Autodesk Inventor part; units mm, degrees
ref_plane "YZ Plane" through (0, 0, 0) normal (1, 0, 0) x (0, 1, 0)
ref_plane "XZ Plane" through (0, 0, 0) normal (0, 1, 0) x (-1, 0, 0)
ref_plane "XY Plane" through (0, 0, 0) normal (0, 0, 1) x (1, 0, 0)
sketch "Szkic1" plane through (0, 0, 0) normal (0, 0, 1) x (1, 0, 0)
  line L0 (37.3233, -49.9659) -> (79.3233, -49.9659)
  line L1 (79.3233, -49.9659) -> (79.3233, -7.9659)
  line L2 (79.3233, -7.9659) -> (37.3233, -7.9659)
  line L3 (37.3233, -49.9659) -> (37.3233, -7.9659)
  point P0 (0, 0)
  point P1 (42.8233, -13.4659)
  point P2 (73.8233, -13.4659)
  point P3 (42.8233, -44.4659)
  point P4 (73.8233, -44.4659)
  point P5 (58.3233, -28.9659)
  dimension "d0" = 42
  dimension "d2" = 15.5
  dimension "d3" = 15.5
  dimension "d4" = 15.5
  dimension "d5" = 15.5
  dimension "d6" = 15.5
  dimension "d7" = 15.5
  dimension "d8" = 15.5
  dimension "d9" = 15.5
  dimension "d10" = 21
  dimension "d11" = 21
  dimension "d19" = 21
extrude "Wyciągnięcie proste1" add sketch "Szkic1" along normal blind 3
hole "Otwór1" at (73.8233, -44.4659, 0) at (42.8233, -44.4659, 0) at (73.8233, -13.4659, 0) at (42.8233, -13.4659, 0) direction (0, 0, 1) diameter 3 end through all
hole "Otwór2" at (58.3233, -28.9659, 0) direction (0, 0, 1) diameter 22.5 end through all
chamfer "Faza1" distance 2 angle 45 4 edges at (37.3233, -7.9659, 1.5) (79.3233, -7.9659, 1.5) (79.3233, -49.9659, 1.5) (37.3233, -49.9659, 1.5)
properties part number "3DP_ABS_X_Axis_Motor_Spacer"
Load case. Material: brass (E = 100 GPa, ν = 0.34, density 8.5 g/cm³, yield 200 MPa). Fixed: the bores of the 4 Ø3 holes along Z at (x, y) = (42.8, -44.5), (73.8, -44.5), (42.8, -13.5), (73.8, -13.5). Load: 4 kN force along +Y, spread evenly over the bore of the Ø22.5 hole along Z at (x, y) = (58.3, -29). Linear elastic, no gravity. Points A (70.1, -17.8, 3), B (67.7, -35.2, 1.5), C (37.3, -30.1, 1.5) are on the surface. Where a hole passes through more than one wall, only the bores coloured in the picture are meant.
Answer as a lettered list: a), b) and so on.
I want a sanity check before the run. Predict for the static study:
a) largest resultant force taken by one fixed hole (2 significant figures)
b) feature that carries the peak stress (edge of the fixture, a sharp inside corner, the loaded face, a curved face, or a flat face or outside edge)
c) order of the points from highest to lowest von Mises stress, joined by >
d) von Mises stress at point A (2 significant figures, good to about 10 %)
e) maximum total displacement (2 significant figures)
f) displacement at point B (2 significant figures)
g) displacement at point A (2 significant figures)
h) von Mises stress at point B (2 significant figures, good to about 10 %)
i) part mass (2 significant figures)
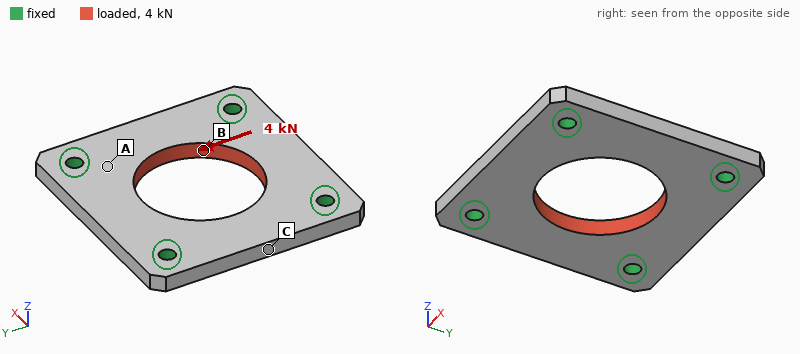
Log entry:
a) 1.0 kN
b) edge of the fixture
c) B > A > C
d) 30 MPa
e) 8.9 µm
f) 4.8 µm
g) 2.8 µm
h) 47 MPa
i) 34 g
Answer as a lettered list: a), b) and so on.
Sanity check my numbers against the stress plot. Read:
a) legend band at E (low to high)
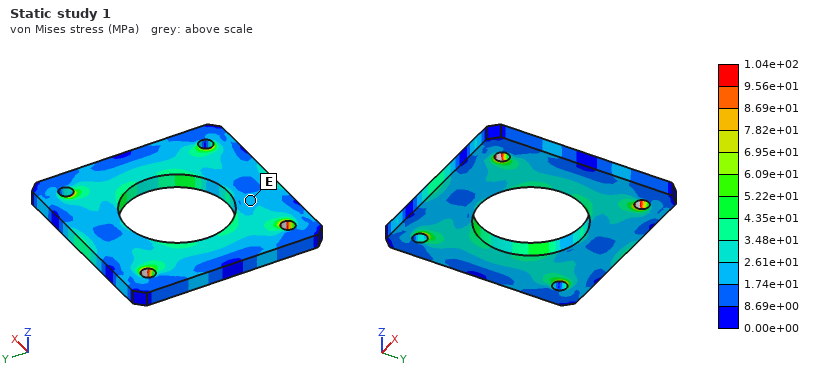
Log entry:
a) 1.74e+01 to 2.61e+01 MPa
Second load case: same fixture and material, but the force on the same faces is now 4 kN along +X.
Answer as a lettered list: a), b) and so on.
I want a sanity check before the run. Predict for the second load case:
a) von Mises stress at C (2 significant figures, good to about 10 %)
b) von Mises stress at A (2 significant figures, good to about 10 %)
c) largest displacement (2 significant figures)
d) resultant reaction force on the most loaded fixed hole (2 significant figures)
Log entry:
a) 39 MPa
b) 30 MPa
c) 8.9 µm
d) 1.0 kN
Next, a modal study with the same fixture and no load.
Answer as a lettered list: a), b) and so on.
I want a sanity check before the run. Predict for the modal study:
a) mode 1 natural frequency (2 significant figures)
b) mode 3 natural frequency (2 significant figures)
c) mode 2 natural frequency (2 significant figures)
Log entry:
a) 11 kHz
b) 11 kHz
c) 11 kHz
